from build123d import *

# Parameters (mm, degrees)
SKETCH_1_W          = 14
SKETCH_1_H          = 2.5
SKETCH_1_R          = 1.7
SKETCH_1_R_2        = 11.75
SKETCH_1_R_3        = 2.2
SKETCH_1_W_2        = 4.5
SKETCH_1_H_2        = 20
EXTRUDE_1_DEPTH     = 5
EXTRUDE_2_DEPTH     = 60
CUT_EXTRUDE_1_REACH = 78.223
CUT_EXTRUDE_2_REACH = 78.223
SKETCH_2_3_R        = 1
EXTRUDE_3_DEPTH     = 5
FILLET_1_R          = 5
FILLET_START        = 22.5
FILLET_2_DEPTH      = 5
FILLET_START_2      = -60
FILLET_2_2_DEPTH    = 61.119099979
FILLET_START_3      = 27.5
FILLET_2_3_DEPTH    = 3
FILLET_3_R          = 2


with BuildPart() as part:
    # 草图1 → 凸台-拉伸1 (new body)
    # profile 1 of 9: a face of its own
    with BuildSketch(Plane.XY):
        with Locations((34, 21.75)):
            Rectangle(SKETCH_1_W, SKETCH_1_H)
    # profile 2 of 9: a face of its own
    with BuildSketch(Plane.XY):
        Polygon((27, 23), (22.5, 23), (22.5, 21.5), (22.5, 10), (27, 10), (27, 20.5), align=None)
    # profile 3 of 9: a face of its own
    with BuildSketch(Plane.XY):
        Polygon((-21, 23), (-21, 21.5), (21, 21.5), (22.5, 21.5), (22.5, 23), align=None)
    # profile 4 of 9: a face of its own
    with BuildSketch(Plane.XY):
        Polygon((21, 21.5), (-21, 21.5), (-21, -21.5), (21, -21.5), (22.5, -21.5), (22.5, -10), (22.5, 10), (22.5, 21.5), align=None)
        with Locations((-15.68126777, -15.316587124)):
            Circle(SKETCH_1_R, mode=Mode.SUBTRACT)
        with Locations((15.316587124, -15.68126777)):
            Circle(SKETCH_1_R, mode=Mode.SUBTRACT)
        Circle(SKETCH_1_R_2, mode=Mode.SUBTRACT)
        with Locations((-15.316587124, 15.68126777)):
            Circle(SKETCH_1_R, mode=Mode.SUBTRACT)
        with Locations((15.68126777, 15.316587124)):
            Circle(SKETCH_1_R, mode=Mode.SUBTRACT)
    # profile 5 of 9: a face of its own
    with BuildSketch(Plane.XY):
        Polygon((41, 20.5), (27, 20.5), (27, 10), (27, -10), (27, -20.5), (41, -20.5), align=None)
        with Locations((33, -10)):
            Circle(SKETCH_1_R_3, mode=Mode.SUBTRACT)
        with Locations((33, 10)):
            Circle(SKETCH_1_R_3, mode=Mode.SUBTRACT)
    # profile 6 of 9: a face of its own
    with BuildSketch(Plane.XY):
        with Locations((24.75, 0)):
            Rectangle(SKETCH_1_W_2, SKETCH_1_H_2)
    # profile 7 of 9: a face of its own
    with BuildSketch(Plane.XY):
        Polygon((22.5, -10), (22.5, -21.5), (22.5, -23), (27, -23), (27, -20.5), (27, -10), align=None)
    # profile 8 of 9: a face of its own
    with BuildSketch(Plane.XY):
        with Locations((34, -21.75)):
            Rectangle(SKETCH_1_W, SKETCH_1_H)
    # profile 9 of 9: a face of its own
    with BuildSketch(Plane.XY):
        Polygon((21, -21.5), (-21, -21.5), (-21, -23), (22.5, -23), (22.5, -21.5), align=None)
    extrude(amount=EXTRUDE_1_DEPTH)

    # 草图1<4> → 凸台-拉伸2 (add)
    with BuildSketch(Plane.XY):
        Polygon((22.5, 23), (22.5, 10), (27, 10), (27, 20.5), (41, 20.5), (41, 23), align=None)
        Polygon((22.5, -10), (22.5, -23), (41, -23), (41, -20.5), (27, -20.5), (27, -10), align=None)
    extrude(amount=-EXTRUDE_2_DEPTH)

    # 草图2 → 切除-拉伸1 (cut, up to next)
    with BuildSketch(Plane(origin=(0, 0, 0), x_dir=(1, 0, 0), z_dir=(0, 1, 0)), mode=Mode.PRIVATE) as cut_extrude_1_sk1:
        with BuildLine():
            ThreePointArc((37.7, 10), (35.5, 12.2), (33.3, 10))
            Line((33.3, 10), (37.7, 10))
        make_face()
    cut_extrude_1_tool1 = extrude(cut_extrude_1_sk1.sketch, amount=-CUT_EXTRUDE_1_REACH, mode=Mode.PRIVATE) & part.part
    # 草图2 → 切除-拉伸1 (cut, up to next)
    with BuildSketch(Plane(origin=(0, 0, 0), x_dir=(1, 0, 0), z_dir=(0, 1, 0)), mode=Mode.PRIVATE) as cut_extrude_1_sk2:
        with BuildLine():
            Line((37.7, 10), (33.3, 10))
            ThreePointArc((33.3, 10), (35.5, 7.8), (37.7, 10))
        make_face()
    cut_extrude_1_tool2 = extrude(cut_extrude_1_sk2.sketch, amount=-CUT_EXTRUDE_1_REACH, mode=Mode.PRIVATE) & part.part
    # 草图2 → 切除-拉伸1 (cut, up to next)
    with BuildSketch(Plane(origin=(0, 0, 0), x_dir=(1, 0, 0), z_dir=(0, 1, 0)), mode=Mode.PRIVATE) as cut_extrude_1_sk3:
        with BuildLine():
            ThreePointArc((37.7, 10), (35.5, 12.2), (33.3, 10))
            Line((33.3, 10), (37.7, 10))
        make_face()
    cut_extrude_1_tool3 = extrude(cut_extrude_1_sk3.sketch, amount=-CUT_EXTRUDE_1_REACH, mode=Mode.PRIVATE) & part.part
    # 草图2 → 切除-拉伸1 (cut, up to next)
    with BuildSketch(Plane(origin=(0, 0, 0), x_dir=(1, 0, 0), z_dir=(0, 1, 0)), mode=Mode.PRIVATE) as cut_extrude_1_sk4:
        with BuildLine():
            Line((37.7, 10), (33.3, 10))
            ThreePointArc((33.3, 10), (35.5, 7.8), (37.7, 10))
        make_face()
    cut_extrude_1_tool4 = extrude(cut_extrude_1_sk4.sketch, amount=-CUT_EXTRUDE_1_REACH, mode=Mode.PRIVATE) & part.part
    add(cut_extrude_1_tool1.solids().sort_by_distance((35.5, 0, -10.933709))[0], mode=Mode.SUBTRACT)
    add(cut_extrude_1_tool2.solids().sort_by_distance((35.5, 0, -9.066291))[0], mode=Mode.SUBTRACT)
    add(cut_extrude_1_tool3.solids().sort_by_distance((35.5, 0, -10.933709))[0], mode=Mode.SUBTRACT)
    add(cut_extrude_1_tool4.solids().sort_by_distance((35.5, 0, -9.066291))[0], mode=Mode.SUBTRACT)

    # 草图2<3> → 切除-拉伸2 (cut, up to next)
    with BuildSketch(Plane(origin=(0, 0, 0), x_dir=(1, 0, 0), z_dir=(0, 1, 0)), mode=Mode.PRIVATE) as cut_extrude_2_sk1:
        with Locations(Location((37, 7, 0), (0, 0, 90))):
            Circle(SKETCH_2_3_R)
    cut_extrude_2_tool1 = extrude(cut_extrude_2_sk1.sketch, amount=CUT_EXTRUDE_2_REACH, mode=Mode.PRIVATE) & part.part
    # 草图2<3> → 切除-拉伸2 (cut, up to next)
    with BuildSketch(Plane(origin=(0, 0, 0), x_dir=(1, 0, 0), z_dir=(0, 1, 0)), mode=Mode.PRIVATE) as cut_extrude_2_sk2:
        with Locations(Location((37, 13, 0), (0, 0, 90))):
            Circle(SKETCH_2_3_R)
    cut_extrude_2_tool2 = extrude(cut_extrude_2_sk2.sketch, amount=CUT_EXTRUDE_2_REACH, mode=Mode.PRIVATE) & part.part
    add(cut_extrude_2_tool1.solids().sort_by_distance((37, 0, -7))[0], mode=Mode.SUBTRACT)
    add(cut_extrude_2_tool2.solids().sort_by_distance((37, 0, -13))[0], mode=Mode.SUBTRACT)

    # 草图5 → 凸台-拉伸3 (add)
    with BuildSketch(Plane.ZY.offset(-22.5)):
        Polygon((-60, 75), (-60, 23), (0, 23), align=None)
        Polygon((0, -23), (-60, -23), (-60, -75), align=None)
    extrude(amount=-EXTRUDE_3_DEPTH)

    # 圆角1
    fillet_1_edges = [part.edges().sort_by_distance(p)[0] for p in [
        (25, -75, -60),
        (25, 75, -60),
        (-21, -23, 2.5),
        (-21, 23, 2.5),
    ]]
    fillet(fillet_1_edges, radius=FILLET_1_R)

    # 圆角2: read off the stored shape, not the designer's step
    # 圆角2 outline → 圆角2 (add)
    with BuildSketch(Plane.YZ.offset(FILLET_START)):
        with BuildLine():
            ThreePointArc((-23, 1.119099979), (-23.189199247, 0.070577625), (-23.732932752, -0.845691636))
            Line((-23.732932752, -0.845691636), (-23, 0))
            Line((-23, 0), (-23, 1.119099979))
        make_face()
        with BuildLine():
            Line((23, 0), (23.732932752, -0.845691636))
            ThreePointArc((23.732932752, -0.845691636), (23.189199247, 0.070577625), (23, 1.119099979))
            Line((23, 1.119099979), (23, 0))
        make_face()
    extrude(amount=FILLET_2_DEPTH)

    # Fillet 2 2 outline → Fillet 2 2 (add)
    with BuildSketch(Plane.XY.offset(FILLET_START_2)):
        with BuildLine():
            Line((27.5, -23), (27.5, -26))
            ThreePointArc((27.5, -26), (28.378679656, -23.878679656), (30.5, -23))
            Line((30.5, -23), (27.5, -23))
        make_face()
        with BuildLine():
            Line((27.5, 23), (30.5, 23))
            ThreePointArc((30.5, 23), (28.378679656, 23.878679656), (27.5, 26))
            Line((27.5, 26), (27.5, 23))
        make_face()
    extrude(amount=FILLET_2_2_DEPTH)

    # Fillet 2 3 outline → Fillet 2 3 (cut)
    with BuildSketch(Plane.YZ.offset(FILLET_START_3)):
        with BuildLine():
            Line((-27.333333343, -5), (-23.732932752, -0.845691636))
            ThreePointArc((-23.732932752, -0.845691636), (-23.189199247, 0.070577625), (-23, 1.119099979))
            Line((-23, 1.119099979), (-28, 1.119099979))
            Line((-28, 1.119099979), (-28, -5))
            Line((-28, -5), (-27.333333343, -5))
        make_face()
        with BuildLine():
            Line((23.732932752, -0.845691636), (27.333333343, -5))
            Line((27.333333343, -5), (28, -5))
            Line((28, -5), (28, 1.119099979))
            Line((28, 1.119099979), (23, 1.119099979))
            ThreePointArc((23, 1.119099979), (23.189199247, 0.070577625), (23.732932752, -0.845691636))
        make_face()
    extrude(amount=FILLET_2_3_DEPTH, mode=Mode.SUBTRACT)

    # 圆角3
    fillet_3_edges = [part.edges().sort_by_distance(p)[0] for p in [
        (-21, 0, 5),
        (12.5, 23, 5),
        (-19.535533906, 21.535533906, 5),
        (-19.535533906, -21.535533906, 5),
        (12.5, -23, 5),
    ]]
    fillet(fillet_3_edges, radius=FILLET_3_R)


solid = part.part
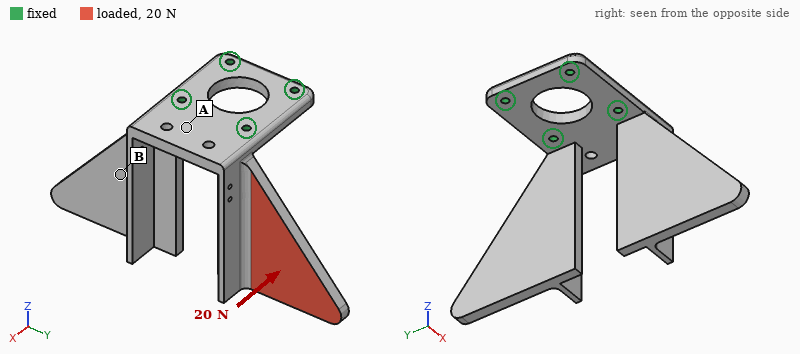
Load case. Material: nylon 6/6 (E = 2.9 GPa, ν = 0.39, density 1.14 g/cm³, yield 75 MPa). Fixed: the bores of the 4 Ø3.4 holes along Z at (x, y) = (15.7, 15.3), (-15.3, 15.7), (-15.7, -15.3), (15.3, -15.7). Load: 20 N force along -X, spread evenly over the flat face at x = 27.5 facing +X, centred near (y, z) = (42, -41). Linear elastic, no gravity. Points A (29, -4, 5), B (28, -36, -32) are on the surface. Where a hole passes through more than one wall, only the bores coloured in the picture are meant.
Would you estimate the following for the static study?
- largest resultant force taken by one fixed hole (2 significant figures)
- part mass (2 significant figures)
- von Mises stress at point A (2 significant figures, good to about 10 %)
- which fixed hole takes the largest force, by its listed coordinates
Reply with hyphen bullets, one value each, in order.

- 32 N
- 44 g
- 2.7 MPa
- (15.7, 15.3)
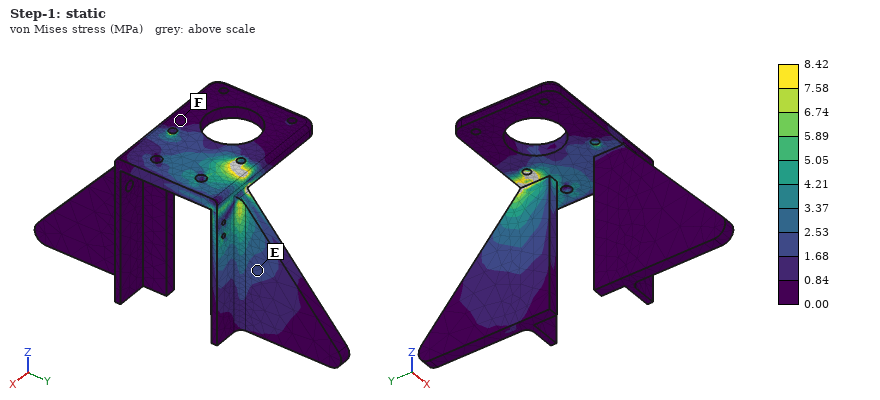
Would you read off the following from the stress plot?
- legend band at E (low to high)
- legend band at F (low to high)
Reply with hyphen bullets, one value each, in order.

- 1.68 to 2.53 MPa
- 0.00 to 0.84 MPa
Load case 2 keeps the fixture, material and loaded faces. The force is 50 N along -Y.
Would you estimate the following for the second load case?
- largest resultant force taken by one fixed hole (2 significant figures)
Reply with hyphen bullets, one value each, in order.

- 56 N
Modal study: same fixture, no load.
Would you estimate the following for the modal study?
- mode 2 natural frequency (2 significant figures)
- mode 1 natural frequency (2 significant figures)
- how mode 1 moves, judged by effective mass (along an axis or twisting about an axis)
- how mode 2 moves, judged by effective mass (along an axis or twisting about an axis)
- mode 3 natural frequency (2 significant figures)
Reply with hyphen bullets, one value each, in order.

- 220 Hz
- 190 Hz
- along X
- twisting about Z
- 280 Hz
